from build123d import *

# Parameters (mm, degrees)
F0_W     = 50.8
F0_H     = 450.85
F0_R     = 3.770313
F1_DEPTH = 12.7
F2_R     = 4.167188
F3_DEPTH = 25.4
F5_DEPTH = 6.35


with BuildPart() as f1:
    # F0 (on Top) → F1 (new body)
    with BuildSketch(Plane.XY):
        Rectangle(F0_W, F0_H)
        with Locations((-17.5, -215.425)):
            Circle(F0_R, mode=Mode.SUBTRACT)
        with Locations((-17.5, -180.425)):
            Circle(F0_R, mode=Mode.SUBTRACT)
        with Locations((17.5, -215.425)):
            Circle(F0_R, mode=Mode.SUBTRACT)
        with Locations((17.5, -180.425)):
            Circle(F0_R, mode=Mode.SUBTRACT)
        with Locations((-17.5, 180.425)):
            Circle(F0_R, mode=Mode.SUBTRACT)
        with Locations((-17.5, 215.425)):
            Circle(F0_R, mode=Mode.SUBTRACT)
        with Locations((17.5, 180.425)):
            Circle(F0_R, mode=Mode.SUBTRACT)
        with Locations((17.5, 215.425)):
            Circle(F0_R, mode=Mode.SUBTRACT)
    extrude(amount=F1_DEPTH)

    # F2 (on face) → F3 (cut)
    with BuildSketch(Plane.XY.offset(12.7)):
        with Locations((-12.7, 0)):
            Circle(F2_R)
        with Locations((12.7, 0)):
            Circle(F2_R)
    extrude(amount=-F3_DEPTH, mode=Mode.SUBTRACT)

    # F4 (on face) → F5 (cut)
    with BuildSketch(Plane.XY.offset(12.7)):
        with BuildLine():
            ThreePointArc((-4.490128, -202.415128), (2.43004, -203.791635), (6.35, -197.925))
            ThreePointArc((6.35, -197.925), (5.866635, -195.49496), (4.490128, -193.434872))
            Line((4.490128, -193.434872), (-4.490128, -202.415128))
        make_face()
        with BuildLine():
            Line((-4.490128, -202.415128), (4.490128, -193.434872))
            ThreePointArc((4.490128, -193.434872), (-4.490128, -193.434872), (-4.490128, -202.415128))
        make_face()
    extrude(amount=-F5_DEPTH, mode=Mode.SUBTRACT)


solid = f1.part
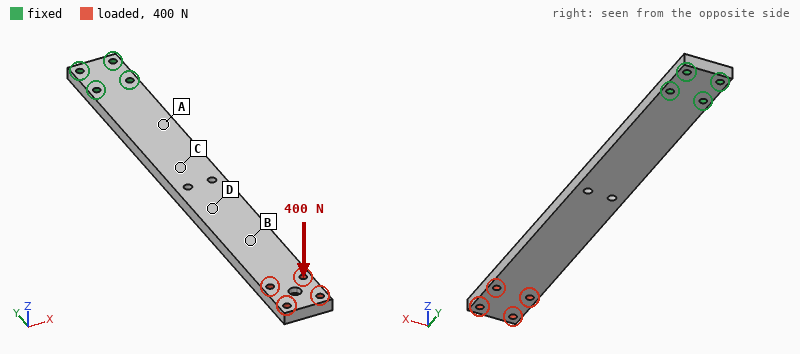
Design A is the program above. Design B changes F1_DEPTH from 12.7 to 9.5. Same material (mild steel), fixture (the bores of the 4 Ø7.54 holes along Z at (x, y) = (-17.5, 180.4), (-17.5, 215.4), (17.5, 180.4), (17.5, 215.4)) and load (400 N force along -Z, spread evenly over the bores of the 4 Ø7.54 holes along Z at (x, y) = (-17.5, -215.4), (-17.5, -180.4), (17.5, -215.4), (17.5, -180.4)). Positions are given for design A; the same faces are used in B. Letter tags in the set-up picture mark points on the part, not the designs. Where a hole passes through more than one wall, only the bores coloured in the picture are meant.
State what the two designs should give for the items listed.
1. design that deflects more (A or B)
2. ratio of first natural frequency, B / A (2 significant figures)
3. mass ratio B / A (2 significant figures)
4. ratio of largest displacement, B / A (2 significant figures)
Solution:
B
0.75
0.75
2.4
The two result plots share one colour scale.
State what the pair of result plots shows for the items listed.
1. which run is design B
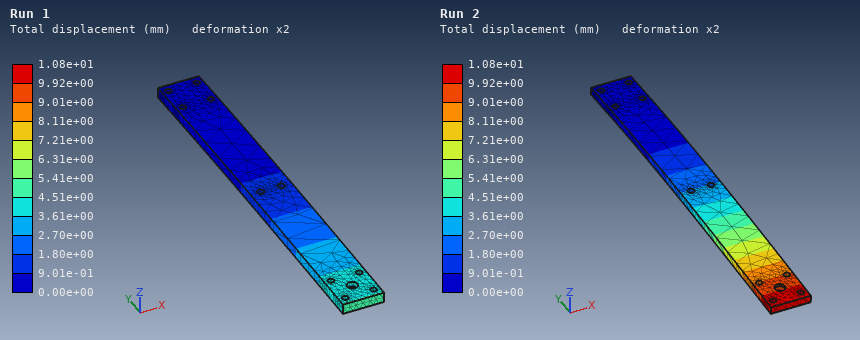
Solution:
Run 2
